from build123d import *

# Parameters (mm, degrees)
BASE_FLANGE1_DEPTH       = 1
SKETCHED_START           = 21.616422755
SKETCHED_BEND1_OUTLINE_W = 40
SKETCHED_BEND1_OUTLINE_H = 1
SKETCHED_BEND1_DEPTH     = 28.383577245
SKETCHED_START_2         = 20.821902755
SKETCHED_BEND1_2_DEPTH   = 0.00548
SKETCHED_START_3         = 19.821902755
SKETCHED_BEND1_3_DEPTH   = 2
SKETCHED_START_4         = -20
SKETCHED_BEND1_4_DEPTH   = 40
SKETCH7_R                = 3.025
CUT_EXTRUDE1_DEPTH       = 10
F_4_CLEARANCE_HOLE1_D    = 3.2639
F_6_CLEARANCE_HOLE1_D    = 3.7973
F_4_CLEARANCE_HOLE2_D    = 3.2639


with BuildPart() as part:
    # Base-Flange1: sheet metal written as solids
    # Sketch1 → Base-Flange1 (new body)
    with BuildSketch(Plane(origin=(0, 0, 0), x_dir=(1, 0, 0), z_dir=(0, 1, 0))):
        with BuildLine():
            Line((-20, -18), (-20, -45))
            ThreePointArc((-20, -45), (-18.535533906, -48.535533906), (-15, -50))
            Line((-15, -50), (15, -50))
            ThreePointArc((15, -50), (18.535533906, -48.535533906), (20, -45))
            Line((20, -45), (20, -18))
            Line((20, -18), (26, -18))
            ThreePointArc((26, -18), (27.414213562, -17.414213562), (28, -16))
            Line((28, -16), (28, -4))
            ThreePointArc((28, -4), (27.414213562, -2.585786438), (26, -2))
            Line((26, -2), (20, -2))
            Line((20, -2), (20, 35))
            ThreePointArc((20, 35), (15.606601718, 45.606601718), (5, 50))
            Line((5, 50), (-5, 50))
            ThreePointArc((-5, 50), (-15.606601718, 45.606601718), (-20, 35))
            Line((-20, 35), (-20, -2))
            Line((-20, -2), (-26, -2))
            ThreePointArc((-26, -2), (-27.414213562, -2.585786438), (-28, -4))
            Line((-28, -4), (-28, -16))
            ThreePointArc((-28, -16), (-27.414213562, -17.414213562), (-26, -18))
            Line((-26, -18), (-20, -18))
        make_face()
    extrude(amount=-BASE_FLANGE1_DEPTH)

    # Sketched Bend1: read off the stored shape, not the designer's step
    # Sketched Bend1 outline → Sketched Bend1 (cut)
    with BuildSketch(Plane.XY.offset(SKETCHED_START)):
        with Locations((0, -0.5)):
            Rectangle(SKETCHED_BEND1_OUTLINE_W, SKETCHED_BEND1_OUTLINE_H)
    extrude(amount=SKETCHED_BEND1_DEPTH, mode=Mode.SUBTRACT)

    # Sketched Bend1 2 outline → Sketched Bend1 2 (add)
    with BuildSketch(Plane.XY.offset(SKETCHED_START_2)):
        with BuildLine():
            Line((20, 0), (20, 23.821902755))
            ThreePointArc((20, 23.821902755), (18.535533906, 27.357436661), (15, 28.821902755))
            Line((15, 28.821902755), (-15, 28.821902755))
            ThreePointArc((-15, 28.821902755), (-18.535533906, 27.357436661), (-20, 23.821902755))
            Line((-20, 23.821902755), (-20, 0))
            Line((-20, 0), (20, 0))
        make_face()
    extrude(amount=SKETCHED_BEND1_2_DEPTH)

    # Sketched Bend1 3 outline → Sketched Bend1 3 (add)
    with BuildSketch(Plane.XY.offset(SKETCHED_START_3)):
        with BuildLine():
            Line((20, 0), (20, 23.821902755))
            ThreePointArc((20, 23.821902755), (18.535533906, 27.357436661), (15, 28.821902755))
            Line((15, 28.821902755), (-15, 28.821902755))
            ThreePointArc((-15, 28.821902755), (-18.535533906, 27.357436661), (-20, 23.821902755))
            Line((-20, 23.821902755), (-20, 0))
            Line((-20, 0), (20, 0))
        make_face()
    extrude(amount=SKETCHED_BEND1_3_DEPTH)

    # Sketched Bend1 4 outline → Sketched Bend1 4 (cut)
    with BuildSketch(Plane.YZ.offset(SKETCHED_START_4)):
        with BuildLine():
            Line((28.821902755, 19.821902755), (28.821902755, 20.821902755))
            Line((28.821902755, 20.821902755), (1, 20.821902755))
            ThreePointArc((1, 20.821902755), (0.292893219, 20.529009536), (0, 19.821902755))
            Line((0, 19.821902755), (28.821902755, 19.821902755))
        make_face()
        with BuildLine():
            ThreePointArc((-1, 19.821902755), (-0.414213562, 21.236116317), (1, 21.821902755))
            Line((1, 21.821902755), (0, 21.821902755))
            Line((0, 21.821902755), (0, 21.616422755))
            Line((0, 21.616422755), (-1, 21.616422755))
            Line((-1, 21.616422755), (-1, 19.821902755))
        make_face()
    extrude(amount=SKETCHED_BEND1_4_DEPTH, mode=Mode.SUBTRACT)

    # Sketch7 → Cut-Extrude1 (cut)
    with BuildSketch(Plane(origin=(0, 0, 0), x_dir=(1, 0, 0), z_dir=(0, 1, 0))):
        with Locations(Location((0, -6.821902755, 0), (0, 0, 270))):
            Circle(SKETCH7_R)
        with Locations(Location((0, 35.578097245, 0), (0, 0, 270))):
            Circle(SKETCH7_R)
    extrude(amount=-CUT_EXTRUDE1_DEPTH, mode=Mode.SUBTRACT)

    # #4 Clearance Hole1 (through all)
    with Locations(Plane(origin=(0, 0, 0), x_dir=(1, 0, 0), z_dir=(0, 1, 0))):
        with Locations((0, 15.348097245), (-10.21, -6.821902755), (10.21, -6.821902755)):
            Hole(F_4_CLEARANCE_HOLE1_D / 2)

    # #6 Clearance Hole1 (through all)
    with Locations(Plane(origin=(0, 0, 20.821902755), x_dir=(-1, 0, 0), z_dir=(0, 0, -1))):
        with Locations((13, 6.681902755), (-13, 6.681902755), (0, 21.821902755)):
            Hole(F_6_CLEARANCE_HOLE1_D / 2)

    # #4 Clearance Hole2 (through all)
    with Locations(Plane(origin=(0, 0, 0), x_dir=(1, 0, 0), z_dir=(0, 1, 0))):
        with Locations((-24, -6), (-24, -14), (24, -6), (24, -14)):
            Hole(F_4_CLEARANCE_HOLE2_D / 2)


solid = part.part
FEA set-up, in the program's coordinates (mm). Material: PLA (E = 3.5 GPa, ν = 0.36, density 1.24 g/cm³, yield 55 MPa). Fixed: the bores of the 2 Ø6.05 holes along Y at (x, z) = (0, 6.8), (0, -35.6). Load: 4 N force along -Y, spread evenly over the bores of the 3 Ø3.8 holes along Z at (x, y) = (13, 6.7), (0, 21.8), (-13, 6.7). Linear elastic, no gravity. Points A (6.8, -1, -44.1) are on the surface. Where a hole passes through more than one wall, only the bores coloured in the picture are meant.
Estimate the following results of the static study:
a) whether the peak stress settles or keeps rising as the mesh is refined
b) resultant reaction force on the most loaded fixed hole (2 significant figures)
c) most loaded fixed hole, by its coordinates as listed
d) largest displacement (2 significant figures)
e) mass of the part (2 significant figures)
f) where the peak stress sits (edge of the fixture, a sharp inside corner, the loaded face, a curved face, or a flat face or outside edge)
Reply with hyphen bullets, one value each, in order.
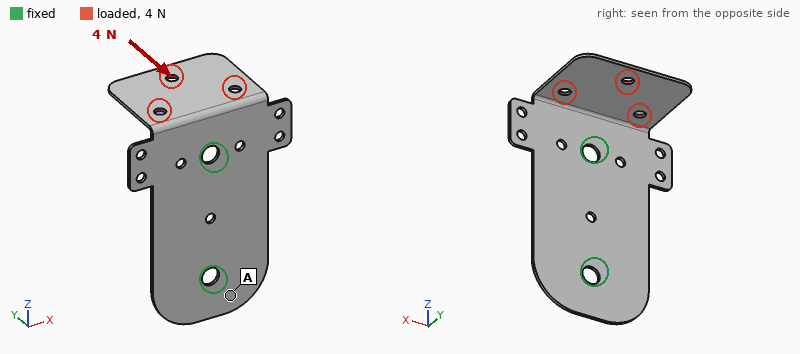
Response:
- keeps rising
- 4.2 N
- (0, 6.8)
- 0.96 mm
- 5.0 g
- edge of the fixture
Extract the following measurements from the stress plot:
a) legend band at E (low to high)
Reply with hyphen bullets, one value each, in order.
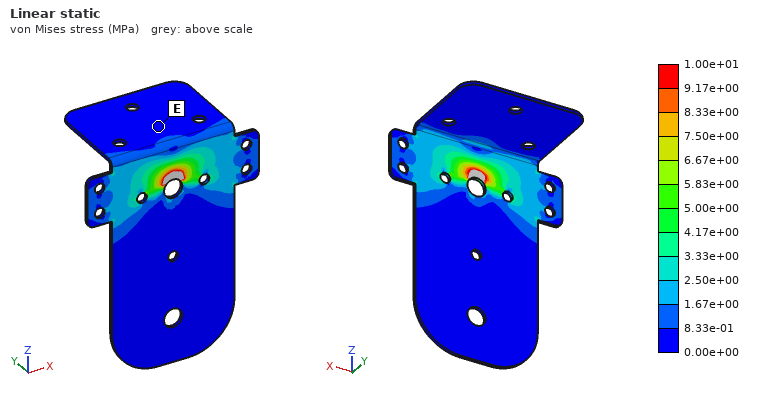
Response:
- 0.00e+00 to 8.33e-01 MPa
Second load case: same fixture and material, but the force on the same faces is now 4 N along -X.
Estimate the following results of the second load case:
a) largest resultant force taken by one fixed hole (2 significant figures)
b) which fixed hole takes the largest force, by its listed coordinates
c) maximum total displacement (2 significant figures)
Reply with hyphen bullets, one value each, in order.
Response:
- 5.0 N
- (0, 6.8)
- 0.96 mm
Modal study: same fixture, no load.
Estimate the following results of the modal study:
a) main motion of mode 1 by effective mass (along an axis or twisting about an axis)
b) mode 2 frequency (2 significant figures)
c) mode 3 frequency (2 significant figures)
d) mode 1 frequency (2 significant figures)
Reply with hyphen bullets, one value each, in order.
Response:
- along Z
- 250 Hz
- 540 Hz
- 190 Hz
